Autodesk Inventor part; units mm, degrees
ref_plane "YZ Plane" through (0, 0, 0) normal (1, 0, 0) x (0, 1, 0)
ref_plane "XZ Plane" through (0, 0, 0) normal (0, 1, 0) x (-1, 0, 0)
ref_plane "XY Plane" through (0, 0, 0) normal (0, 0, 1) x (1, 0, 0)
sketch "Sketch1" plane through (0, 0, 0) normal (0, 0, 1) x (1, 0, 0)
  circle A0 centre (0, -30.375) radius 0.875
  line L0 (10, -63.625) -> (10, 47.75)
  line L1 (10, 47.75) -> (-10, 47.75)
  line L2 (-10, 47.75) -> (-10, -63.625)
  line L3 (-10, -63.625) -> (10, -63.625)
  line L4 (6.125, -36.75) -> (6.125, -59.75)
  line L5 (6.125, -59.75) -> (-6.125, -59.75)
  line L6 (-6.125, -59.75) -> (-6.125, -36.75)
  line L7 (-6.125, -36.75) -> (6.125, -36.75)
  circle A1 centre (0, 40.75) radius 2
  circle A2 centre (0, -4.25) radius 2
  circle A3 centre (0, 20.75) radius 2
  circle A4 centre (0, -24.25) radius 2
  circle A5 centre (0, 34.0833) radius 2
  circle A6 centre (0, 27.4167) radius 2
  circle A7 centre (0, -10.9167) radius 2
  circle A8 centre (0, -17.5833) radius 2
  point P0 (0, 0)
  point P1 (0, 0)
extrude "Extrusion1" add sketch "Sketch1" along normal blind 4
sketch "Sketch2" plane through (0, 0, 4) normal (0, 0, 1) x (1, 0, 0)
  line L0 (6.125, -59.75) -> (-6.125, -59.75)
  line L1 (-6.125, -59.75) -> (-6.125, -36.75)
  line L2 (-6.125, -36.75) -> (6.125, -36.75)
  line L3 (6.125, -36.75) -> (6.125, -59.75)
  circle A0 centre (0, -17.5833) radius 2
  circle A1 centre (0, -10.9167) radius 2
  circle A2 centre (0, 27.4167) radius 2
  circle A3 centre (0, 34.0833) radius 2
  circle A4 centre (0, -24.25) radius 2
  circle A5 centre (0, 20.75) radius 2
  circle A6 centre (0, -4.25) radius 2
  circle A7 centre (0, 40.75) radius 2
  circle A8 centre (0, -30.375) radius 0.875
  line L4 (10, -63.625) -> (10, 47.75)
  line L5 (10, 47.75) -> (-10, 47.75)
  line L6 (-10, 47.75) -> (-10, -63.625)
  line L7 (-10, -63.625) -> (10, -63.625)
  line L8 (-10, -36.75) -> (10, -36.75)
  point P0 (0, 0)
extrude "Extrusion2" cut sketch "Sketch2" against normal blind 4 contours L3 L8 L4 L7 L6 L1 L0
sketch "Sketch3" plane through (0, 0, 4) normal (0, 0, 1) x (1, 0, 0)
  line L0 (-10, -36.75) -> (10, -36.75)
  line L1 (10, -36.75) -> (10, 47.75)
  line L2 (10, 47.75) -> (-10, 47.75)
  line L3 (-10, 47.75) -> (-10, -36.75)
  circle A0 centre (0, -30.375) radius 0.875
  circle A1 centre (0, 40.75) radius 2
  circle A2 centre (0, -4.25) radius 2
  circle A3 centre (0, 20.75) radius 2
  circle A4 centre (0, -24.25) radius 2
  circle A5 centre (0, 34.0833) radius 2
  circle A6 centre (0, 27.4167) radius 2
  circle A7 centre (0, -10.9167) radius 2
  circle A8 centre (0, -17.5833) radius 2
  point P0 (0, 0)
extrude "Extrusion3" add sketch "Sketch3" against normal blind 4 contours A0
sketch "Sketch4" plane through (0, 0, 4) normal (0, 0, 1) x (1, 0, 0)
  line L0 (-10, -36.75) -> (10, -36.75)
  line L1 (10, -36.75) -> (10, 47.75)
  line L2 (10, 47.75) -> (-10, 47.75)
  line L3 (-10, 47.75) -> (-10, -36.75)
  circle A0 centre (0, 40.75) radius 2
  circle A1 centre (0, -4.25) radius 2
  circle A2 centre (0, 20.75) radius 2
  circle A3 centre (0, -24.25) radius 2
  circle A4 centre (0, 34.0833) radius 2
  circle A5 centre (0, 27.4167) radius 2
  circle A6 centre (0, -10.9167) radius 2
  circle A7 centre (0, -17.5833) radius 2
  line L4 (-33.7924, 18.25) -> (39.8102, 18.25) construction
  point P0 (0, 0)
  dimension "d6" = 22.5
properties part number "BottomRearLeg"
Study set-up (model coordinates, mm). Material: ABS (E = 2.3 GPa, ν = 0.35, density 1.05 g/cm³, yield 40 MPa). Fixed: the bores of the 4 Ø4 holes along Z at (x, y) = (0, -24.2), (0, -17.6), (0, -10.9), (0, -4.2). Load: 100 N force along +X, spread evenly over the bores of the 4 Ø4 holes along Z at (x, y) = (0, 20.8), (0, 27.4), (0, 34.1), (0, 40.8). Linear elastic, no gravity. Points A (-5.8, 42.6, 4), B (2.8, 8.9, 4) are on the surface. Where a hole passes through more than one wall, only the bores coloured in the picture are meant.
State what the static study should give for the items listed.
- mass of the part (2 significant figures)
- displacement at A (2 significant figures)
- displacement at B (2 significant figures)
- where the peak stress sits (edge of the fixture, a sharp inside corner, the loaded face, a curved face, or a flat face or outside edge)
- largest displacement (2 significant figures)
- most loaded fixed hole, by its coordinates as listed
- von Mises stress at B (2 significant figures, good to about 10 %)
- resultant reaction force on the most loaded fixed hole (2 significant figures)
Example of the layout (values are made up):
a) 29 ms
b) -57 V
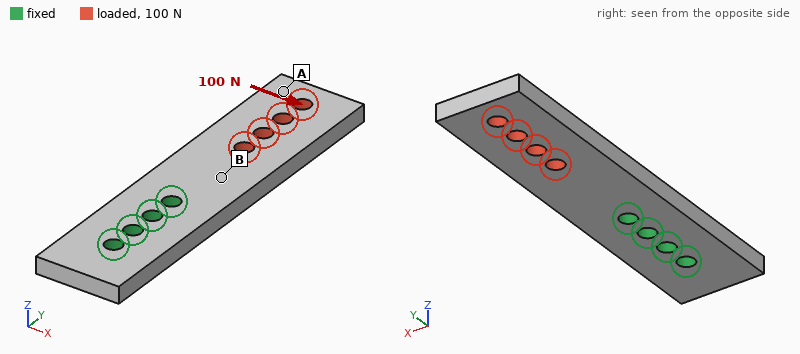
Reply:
a) 6.7 g
b) 0.66 mm
c) 0.13 mm
d) edge of the fixture
e) 0.75 mm
f) (0, -4.2)
g) 3.7 MPa
h) 270 N
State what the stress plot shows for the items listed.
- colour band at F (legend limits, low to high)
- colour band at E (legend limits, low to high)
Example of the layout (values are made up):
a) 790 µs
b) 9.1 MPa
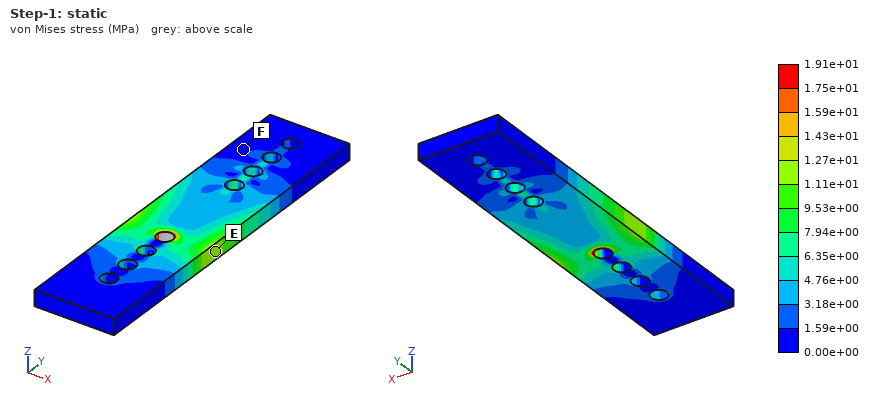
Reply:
a) 0.00e+00 to 1.59e+00 MPa
b) 1.11e+01 to 1.27e+01 MPa
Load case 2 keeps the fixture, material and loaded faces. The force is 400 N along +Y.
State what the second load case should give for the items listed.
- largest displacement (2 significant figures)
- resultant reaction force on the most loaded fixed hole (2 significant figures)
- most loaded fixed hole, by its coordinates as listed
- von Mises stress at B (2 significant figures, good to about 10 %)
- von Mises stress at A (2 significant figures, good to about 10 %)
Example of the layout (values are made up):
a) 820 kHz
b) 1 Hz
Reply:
a) 98 µm
b) 280 N
c) (0, -4.2)
d) 5.4 MPa
e) 1.5 MPa
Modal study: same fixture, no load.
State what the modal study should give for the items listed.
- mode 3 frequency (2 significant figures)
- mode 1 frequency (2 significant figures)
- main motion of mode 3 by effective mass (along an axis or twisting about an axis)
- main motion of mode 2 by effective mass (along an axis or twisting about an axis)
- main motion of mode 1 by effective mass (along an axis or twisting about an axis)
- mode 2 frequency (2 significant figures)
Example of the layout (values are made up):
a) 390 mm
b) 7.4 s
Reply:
a) 1600 Hz
b) 370 Hz
c) twisting about Y
d) along X
e) along Z
f) 1300 Hz
